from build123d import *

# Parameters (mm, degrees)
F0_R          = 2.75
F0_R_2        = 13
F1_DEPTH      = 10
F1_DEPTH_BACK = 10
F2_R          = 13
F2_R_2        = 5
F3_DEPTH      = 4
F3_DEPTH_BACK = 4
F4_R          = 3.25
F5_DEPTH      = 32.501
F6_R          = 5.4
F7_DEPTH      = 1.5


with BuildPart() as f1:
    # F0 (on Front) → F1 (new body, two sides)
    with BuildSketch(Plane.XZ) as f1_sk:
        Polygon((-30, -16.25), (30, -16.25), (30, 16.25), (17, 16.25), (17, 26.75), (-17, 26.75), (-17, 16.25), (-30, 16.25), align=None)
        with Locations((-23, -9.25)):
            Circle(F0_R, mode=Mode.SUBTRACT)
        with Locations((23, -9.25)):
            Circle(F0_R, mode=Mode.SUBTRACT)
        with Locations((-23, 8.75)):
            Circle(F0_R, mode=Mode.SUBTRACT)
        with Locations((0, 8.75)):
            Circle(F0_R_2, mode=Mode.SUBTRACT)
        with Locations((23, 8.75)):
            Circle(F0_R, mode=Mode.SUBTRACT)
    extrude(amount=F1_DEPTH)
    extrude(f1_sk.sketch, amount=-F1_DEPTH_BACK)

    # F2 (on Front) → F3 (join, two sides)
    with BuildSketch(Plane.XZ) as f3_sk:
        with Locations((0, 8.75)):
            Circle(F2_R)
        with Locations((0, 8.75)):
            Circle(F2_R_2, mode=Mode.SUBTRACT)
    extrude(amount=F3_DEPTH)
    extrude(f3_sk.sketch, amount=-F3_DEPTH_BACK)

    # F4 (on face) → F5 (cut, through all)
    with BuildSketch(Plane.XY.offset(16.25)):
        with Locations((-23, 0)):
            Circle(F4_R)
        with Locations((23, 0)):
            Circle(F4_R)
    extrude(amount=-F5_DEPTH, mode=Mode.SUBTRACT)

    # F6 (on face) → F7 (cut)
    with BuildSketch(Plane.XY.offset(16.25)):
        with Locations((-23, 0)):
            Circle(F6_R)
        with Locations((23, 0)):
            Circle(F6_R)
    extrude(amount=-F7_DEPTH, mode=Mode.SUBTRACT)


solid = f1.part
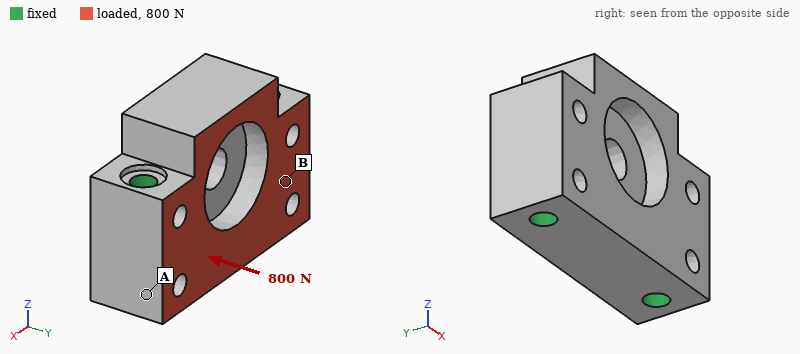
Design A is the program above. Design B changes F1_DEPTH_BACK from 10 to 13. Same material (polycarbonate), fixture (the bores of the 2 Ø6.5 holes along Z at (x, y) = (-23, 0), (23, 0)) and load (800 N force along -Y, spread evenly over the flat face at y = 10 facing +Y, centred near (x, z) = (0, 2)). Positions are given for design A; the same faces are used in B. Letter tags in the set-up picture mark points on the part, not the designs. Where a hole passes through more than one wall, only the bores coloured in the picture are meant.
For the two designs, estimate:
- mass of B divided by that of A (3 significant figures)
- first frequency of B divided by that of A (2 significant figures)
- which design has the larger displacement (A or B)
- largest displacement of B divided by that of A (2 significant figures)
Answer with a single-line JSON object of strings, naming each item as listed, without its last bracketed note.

{"mass of B divided by that of A": "1.14", "first frequency of B divided by that of A": "1.0", "which design has the larger displacement": "A", "largest displacement of B divided by that of A": "0.88"}
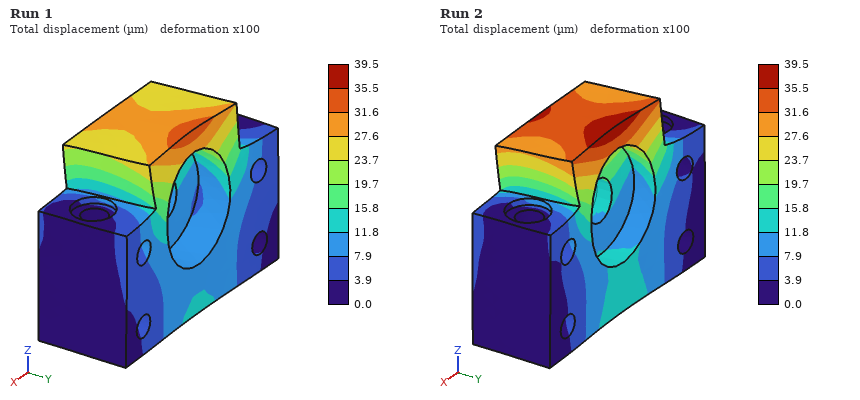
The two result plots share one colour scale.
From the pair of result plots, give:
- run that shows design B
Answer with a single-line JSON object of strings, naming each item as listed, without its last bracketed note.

{"run that shows design B": "Run 1"}
